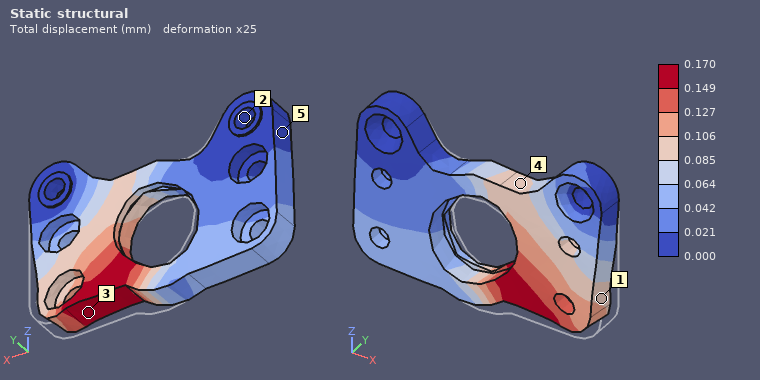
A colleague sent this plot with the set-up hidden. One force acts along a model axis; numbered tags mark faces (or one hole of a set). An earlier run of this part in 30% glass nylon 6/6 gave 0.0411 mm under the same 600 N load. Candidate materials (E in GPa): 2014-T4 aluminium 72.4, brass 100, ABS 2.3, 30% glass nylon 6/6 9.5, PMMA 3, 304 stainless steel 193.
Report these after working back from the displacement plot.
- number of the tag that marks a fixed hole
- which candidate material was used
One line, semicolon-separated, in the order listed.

2; ABS
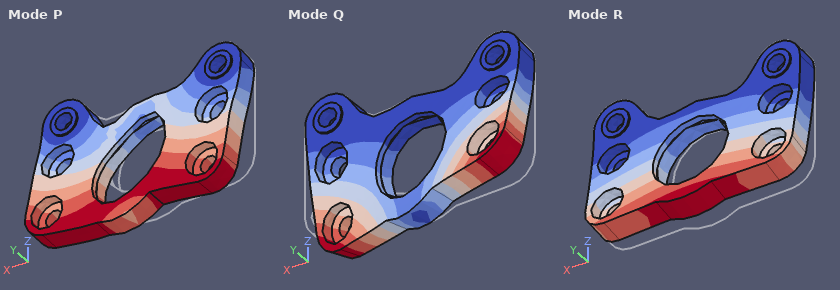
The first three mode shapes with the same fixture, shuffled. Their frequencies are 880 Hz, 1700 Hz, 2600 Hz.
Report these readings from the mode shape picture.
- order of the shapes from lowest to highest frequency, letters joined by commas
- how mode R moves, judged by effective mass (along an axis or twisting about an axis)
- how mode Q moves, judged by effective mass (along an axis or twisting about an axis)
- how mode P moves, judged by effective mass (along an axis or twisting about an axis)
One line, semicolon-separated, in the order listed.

R, Q, P; along Y; twisting about Z; along X
